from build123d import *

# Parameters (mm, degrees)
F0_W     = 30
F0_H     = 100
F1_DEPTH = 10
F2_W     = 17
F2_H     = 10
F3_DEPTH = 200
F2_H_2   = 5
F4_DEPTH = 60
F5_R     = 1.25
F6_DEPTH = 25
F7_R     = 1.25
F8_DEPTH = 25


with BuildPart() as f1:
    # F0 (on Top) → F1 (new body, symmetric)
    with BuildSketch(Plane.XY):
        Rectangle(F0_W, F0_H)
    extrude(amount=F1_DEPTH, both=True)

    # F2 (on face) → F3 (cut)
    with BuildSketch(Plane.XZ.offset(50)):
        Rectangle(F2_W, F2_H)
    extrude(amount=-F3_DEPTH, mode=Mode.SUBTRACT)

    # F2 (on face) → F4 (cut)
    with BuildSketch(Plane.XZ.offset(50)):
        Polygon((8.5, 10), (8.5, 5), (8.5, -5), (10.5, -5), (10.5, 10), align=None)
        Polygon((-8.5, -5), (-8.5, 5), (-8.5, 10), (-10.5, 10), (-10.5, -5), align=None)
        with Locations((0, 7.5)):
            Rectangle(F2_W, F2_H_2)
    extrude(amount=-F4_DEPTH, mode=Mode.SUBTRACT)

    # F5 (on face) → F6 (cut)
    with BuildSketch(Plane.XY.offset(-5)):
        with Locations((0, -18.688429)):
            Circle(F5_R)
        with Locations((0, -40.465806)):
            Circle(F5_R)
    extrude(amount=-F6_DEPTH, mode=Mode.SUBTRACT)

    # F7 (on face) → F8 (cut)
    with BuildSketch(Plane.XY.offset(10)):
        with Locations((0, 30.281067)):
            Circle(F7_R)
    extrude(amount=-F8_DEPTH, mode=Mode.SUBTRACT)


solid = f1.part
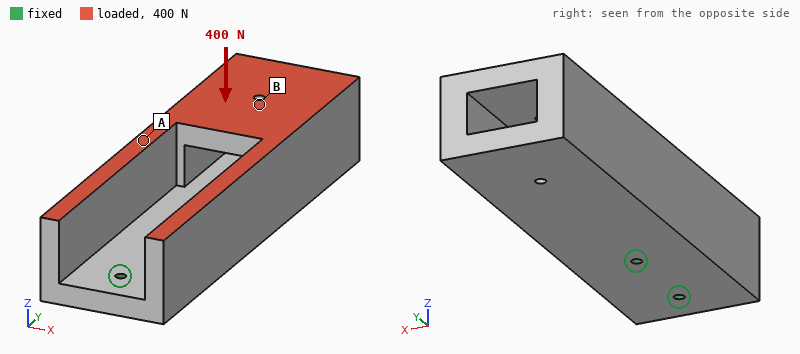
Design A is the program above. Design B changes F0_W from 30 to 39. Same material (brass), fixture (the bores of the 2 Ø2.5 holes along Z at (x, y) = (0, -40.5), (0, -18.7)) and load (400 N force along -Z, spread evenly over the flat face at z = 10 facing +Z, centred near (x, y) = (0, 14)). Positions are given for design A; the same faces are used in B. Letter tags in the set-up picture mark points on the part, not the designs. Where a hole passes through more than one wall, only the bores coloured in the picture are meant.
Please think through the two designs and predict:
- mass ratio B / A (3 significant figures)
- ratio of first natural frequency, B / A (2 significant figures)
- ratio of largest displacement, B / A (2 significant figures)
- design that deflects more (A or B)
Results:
1.53
0.94
0.68
A
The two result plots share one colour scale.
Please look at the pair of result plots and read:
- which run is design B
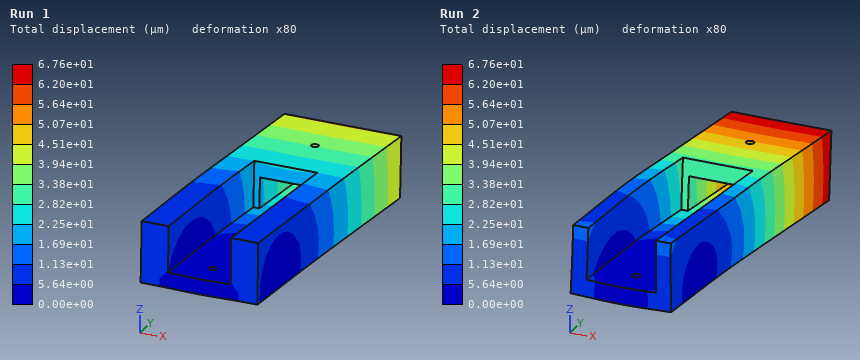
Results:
Run 1
